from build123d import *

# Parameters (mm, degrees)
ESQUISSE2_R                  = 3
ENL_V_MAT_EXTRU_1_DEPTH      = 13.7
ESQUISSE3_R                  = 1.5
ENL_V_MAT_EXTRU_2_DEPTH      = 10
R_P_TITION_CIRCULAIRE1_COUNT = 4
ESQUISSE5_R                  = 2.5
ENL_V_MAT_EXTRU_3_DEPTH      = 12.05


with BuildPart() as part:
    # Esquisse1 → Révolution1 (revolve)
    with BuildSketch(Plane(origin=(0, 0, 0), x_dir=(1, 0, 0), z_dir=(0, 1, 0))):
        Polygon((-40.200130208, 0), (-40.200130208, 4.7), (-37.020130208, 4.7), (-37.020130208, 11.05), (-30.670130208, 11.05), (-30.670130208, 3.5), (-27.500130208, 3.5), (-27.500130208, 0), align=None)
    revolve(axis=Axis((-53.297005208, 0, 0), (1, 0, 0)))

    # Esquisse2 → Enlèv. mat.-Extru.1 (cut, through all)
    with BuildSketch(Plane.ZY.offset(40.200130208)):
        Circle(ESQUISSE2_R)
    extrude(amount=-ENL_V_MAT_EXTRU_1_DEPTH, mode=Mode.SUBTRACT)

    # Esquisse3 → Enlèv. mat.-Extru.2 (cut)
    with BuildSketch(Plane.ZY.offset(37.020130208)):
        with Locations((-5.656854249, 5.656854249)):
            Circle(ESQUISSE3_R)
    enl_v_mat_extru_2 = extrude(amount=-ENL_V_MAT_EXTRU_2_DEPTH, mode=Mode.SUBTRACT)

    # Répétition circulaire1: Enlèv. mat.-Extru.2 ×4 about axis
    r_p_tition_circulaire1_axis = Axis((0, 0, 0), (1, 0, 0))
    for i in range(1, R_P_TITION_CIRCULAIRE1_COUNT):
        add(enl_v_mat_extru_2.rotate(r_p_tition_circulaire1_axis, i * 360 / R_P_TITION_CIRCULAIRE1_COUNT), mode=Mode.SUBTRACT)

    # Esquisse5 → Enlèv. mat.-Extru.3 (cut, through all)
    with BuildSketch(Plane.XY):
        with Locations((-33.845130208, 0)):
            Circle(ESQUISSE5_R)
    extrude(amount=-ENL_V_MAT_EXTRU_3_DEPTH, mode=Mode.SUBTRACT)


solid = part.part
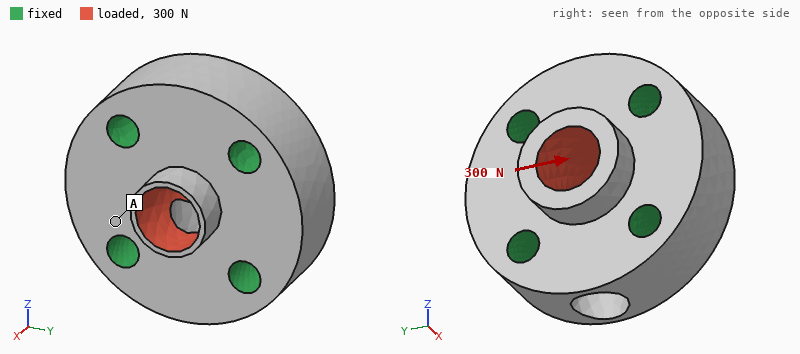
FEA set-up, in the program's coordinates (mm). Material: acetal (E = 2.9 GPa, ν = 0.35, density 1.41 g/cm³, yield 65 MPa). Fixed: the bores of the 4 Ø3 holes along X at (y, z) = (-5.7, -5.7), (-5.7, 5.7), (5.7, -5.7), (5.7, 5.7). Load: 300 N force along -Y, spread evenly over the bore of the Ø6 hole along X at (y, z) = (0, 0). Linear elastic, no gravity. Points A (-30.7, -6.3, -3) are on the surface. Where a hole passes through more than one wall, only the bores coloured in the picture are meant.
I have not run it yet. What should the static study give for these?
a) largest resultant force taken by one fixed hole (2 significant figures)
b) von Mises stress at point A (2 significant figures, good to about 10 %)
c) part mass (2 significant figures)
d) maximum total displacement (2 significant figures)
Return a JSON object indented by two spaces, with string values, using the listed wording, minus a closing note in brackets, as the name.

{
  "largest resultant force taken by one fixed hole": "88 N",
  "von Mises stress at point A": "1.9 MPa",
  "part mass": "2.9 g",
  "maximum total displacement": "49 µm"
}
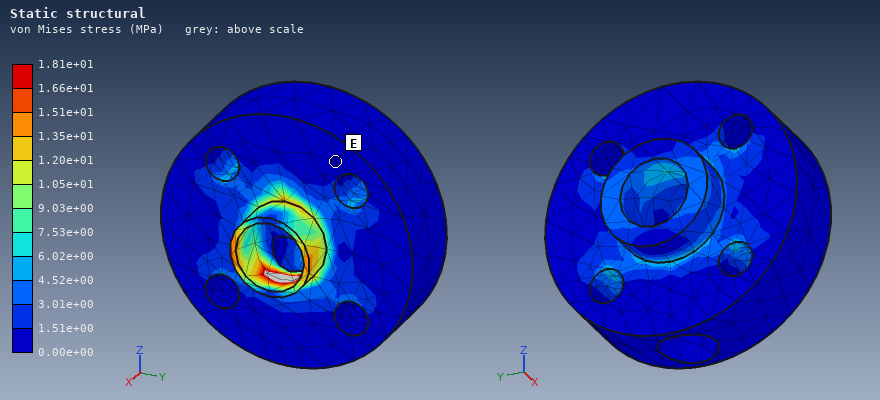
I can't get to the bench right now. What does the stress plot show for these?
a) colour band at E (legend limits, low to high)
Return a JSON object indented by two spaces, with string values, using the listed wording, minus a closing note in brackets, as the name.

{
  "colour band at E": "0.00e+00 to 1.51e+00 MPa"
}
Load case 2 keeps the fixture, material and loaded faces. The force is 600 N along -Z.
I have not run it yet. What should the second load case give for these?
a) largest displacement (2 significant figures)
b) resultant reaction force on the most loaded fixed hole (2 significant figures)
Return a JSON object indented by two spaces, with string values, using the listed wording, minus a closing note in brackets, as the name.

{
  "largest displacement": "0.11 mm",
  "resultant reaction force on the most loaded fixed hole": "170 N"
}
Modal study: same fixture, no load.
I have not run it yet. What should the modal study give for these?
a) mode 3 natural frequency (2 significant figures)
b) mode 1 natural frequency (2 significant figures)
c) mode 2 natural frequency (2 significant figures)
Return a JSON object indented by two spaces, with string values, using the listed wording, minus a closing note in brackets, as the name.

{
  "mode 3 natural frequency": "30 kHz",
  "mode 1 natural frequency": "28 kHz",
  "mode 2 natural frequency": "29 kHz"
}
